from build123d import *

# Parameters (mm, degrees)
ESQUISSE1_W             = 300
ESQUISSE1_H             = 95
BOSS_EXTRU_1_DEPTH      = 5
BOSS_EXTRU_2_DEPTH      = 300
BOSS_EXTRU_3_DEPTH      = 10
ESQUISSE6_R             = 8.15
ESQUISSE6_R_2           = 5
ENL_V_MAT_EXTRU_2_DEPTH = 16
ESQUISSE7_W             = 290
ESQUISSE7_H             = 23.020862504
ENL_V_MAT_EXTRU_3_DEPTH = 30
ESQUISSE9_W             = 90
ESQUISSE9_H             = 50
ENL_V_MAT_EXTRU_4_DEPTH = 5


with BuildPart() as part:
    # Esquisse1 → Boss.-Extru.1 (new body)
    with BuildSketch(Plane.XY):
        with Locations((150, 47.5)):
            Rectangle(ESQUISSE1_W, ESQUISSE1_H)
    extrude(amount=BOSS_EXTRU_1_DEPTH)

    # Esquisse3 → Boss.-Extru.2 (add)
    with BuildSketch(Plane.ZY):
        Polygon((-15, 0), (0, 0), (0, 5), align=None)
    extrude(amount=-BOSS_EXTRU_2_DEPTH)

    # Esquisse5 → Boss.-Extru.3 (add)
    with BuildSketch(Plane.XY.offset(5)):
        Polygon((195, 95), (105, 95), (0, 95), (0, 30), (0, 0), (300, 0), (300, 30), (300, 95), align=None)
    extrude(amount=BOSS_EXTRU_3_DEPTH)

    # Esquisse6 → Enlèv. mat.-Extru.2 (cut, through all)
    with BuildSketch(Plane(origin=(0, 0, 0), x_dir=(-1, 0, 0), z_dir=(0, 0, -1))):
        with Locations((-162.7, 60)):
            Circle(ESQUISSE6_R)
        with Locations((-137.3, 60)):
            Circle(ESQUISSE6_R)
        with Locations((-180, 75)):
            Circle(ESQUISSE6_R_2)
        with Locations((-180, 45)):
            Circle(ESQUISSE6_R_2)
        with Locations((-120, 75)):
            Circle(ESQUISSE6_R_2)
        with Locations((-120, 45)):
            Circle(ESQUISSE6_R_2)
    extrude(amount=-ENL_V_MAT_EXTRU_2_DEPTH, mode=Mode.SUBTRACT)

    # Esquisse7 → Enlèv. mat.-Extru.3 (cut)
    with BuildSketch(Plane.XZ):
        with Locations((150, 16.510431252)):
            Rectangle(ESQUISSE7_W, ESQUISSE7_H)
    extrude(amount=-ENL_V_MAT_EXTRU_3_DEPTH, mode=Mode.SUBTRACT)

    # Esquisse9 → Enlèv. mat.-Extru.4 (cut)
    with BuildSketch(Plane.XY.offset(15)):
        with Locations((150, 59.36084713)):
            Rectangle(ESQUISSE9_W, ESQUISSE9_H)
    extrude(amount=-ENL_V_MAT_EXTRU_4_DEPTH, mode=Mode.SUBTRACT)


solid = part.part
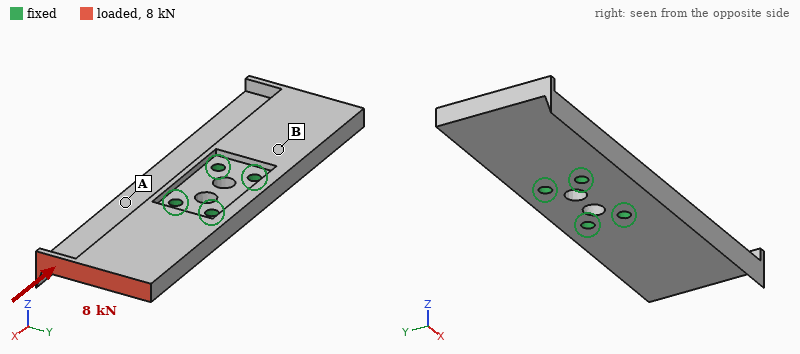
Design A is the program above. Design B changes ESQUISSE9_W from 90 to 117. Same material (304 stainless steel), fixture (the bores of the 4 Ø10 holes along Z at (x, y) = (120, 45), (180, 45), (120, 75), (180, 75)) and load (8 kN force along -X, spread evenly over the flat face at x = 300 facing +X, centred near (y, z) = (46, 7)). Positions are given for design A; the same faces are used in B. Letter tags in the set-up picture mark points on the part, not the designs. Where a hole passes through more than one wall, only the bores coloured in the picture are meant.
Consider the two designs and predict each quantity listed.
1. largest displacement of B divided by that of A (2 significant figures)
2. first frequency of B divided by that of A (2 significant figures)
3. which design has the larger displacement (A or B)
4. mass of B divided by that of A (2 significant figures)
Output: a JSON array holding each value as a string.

["1.2", "0.94", "B", "0.98"]
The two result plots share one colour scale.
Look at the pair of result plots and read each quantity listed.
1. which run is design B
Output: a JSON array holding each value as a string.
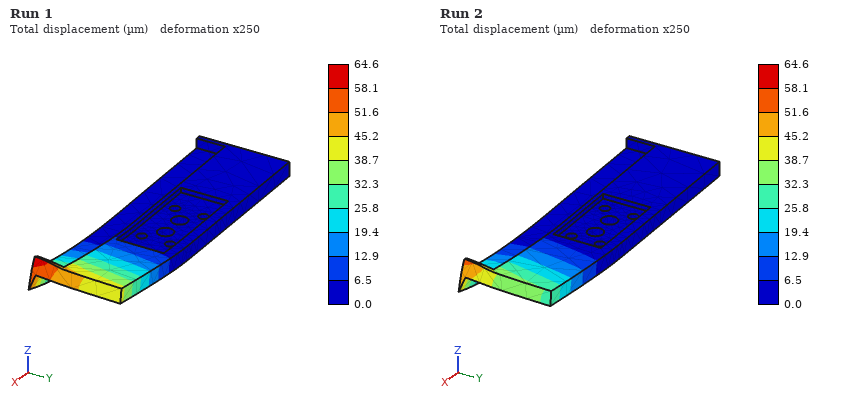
["Run 1"]
